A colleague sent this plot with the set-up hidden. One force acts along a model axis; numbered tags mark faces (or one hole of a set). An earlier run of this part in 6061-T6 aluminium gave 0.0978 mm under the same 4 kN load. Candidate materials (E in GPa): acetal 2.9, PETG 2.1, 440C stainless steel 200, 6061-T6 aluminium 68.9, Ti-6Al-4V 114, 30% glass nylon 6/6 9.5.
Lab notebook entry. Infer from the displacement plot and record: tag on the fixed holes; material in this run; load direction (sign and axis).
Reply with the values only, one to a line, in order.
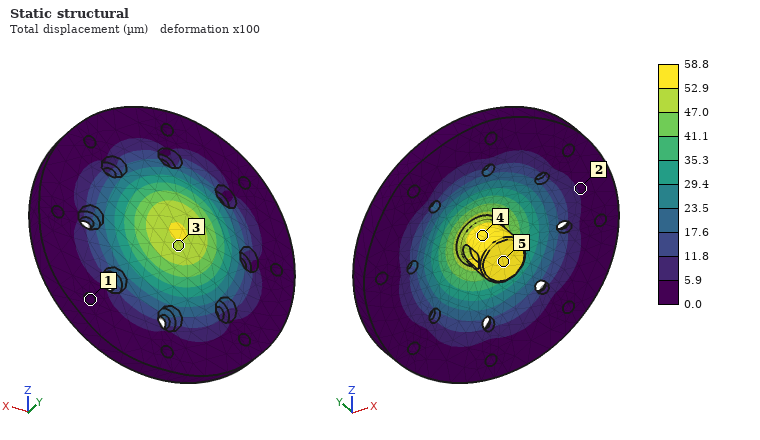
1
Ti-6Al-4V
+Y
